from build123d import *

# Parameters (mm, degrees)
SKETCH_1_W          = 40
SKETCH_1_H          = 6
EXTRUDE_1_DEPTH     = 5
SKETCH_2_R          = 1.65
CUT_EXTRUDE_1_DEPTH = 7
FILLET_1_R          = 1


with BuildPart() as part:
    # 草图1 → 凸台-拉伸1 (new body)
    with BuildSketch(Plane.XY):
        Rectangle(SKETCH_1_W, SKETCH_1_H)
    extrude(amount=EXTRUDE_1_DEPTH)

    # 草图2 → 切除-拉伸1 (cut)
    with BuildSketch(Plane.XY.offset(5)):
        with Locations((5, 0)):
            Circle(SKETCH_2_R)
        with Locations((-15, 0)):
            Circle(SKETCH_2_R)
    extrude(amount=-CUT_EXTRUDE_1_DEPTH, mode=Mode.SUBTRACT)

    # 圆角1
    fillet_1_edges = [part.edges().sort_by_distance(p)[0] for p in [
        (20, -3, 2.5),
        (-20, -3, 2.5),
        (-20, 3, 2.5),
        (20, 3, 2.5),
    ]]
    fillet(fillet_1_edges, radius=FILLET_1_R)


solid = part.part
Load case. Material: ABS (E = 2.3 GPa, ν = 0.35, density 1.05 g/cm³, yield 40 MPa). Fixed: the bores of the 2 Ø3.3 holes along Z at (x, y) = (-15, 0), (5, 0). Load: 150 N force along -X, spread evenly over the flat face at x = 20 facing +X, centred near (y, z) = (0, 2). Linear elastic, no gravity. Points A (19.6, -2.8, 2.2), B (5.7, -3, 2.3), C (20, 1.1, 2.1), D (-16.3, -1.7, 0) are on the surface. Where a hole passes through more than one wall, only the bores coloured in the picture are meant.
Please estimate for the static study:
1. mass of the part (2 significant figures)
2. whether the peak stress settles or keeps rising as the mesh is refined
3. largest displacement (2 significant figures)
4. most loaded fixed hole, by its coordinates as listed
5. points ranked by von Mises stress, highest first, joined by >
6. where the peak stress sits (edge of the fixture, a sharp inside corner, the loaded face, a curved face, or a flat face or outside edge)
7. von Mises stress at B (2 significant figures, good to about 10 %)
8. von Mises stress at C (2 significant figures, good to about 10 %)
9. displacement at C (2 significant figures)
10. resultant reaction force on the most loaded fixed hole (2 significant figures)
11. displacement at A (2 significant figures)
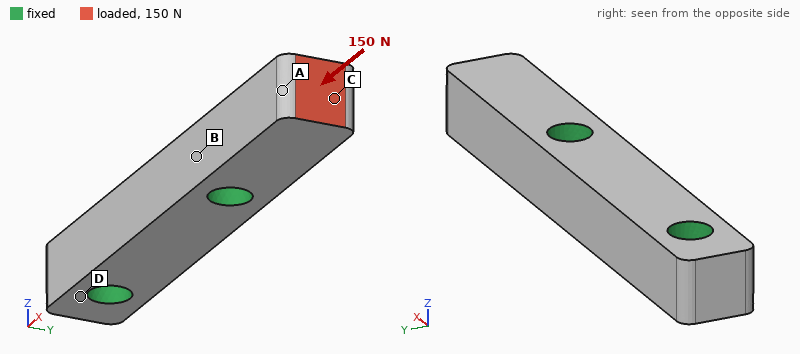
1.2 g
keeps rising
35 µm
(5, 0)
C > B > A > D
edge of the fixture
2.5 MPa
5.3 MPa
33 µm
150 N
26 µm
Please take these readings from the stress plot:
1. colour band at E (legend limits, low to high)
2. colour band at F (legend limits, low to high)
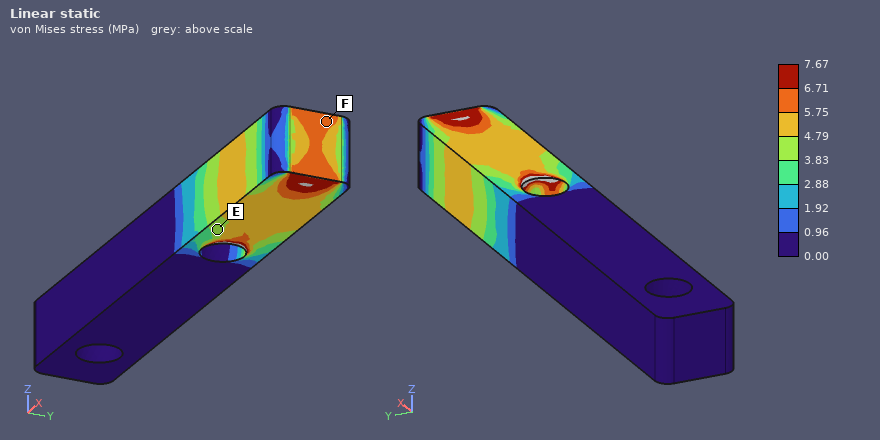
3.83 to 4.79 MPa
5.75 to 6.71 MPa
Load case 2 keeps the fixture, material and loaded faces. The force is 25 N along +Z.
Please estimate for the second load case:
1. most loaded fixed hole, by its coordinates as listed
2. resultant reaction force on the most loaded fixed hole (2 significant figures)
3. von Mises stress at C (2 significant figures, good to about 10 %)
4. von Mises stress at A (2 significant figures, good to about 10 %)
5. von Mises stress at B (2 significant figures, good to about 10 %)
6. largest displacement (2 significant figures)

(5, 0)
25 N
2.5 MPa
1.6 MPa
3.1 MPa
0.18 mm
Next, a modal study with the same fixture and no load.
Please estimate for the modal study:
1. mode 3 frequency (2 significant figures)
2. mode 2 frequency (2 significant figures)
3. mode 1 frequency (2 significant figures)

15 kHz
5800 Hz
5700 Hz
